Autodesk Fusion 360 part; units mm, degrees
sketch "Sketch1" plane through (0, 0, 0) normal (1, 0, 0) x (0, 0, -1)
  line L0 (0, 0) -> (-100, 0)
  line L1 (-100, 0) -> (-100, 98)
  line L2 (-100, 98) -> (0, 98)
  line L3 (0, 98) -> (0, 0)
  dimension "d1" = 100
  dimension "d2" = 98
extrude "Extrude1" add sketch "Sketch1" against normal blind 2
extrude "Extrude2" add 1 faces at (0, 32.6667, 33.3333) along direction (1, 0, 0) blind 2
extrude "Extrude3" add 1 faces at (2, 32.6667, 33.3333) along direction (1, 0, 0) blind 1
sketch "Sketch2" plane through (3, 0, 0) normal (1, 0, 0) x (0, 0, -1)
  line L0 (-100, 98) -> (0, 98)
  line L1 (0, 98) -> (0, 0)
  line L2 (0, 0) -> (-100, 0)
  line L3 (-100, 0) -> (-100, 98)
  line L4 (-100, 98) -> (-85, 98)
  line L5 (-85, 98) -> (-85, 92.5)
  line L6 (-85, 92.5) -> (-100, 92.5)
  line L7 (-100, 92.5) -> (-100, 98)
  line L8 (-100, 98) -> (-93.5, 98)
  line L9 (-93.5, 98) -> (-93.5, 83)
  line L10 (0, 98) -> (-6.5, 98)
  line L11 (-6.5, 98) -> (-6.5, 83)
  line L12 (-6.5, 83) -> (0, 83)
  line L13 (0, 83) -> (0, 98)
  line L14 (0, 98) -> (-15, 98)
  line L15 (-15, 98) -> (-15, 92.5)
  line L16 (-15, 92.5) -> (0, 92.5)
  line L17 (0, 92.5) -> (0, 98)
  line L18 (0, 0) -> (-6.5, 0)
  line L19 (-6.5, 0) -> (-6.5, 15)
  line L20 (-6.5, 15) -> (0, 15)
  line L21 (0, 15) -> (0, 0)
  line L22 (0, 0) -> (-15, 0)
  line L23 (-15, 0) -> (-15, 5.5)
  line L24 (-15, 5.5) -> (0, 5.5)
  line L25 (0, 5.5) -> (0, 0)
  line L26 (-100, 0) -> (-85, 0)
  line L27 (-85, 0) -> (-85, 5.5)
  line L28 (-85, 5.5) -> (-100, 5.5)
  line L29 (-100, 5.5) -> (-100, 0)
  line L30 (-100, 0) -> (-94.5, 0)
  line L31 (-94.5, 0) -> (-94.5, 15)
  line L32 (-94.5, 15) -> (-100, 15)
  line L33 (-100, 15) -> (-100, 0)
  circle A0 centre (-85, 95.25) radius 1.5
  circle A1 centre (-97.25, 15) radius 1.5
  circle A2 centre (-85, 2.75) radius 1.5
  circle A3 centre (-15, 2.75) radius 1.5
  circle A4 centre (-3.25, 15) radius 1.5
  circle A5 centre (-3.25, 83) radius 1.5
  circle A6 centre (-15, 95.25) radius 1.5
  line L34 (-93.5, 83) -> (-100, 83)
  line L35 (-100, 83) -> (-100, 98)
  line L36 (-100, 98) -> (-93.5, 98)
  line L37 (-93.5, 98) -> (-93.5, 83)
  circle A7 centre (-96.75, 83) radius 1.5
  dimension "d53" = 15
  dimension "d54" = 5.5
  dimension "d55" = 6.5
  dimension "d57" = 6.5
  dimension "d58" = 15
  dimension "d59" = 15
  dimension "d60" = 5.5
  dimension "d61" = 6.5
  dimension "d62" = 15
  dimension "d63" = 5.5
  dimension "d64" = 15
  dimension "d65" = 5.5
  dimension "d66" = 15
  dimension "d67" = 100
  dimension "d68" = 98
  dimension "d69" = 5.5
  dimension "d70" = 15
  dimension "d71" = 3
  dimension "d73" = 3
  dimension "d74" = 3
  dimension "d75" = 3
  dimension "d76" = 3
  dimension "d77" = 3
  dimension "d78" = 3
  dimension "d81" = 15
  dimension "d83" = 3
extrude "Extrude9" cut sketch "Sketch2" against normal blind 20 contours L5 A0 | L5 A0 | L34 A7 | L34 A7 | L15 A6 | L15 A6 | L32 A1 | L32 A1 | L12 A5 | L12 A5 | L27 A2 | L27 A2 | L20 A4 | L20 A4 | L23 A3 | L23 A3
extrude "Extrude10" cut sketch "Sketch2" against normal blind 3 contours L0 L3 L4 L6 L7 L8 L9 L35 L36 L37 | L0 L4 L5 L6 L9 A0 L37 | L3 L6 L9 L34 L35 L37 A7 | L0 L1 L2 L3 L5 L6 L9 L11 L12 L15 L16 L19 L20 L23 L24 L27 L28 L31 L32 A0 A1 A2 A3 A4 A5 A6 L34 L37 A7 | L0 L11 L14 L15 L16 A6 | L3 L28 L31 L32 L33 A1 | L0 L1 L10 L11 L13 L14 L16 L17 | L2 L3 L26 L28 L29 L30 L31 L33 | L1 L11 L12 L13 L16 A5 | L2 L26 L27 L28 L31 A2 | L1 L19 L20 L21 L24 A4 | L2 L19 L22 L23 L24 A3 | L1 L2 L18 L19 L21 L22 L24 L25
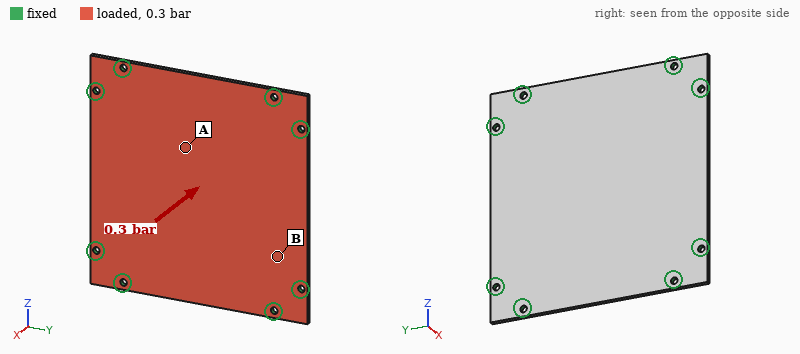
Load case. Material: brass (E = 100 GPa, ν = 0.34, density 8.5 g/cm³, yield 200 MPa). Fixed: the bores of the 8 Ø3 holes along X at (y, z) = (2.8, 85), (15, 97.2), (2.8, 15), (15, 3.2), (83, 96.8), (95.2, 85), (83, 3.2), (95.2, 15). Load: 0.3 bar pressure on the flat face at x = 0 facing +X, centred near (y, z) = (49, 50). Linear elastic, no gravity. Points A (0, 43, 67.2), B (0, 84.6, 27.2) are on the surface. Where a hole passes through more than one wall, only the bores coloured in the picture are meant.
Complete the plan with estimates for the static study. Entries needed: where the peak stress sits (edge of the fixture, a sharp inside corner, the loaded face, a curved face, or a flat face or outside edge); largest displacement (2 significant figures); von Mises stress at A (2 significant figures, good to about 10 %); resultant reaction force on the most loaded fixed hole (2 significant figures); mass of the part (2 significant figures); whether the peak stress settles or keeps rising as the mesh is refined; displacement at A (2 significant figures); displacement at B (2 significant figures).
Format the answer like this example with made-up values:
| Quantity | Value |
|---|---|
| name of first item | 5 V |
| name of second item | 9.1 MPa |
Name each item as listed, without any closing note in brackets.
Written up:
| Quantity | Value |
|---|---|
| where the peak stress sits | edge of the fixture |
| largest displacement | 0.12 mm |
| von Mises stress at A | 14 MPa |
| resultant reaction force on the most loaded fixed hole | 38 N |
| mass of the part | 170 g |
| whether the peak stress settles or keeps rising as the mesh is refined | keeps rising |
| displacement at A | 0.099 mm |
| displacement at B | 0.036 mm |
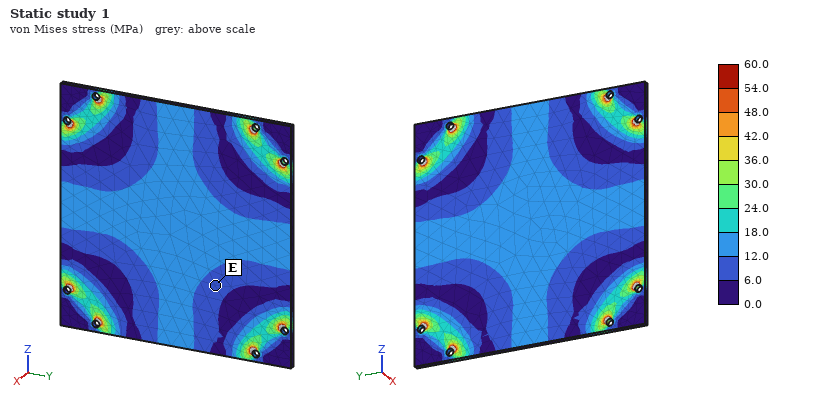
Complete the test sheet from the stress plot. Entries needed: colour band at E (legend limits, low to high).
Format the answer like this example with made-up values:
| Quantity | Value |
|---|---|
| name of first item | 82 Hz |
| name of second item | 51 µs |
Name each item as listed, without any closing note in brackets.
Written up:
| Quantity | Value |
|---|---|
| colour band at E | 6.0 to 12.0 MPa |
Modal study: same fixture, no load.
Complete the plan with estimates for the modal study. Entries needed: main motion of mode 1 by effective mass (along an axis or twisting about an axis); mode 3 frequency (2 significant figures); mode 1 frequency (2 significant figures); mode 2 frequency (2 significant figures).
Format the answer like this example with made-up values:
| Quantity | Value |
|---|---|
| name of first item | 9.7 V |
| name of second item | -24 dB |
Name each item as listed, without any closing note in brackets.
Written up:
| Quantity | Value |
|---|---|
| main motion of mode 1 by effective mass | along X |
| mode 3 frequency | 1500 Hz |
| mode 1 frequency | 770 Hz |
| mode 2 frequency | 1400 Hz |
